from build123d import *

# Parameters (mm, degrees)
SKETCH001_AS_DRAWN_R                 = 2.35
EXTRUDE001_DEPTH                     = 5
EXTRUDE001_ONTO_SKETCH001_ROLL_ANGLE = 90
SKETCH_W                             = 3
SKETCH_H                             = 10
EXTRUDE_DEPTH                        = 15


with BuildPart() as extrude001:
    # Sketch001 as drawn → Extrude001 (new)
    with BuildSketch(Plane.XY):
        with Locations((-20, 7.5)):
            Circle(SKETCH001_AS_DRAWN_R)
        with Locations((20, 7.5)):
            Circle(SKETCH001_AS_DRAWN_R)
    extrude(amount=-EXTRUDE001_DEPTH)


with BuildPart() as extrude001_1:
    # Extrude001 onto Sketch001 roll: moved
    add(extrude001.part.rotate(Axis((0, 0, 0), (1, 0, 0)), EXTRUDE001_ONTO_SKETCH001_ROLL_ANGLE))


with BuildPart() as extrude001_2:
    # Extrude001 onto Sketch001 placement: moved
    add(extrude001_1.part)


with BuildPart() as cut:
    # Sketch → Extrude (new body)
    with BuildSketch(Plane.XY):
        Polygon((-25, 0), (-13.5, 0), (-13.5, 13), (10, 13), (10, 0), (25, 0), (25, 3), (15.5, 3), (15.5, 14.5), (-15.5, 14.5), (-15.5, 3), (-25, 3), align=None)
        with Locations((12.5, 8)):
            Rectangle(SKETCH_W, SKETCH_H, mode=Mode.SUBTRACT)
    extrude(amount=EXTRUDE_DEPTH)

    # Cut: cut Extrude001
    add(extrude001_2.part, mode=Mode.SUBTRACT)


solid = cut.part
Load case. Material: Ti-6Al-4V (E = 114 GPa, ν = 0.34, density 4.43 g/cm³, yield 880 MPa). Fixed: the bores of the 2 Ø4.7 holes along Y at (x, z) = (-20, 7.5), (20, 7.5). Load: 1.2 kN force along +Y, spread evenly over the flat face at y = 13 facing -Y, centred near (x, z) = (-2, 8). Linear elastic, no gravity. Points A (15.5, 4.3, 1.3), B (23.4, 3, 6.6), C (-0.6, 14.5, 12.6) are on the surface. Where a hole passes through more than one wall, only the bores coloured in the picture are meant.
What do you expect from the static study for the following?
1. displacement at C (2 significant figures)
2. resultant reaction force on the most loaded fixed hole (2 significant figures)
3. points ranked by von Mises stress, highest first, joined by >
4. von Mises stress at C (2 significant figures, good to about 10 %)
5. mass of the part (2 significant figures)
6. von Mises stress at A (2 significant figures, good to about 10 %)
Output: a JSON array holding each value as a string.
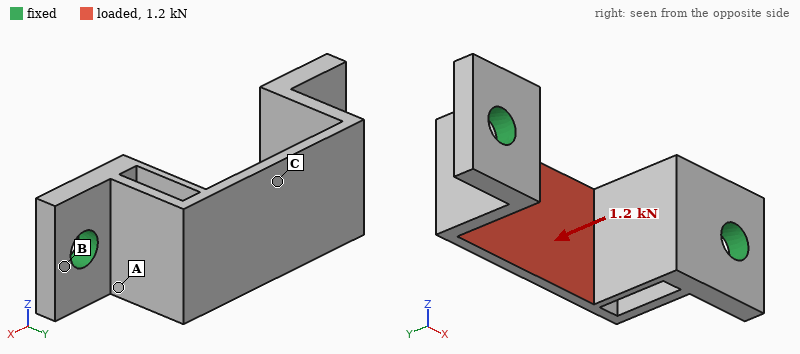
["0.16 mm", "680 N", "C > A > B", "280 MPa", "11 g", "100 MPa"]
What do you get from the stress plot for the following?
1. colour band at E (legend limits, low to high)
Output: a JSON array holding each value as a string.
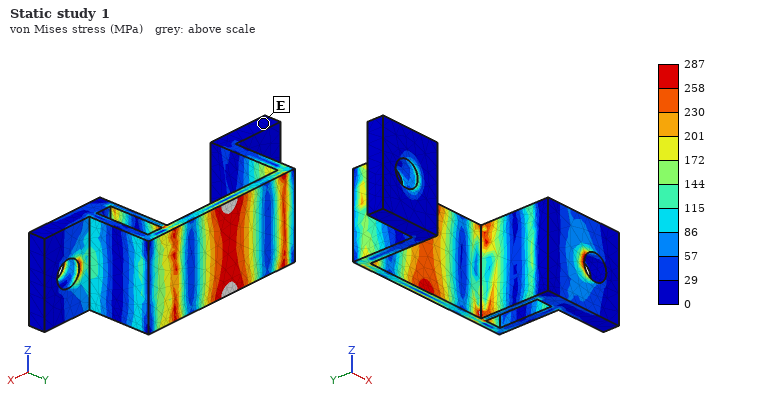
["0 to 29 MPa"]
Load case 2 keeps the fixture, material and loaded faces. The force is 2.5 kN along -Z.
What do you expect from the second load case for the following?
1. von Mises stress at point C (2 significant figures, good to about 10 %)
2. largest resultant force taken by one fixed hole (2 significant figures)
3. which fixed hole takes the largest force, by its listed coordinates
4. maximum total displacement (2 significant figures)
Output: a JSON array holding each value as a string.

["140 MPa", "1.4 kN", "(-20, 7.5)", "0.17 mm"]
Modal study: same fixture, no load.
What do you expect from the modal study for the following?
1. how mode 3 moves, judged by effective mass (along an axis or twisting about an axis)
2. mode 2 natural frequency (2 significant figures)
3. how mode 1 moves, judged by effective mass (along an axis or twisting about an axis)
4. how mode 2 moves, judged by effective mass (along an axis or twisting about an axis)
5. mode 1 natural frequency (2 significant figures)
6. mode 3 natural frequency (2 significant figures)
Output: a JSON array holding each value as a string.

["along Y", "9500 Hz", "along X", "along Z", "6100 Hz", "10 kHz"]
